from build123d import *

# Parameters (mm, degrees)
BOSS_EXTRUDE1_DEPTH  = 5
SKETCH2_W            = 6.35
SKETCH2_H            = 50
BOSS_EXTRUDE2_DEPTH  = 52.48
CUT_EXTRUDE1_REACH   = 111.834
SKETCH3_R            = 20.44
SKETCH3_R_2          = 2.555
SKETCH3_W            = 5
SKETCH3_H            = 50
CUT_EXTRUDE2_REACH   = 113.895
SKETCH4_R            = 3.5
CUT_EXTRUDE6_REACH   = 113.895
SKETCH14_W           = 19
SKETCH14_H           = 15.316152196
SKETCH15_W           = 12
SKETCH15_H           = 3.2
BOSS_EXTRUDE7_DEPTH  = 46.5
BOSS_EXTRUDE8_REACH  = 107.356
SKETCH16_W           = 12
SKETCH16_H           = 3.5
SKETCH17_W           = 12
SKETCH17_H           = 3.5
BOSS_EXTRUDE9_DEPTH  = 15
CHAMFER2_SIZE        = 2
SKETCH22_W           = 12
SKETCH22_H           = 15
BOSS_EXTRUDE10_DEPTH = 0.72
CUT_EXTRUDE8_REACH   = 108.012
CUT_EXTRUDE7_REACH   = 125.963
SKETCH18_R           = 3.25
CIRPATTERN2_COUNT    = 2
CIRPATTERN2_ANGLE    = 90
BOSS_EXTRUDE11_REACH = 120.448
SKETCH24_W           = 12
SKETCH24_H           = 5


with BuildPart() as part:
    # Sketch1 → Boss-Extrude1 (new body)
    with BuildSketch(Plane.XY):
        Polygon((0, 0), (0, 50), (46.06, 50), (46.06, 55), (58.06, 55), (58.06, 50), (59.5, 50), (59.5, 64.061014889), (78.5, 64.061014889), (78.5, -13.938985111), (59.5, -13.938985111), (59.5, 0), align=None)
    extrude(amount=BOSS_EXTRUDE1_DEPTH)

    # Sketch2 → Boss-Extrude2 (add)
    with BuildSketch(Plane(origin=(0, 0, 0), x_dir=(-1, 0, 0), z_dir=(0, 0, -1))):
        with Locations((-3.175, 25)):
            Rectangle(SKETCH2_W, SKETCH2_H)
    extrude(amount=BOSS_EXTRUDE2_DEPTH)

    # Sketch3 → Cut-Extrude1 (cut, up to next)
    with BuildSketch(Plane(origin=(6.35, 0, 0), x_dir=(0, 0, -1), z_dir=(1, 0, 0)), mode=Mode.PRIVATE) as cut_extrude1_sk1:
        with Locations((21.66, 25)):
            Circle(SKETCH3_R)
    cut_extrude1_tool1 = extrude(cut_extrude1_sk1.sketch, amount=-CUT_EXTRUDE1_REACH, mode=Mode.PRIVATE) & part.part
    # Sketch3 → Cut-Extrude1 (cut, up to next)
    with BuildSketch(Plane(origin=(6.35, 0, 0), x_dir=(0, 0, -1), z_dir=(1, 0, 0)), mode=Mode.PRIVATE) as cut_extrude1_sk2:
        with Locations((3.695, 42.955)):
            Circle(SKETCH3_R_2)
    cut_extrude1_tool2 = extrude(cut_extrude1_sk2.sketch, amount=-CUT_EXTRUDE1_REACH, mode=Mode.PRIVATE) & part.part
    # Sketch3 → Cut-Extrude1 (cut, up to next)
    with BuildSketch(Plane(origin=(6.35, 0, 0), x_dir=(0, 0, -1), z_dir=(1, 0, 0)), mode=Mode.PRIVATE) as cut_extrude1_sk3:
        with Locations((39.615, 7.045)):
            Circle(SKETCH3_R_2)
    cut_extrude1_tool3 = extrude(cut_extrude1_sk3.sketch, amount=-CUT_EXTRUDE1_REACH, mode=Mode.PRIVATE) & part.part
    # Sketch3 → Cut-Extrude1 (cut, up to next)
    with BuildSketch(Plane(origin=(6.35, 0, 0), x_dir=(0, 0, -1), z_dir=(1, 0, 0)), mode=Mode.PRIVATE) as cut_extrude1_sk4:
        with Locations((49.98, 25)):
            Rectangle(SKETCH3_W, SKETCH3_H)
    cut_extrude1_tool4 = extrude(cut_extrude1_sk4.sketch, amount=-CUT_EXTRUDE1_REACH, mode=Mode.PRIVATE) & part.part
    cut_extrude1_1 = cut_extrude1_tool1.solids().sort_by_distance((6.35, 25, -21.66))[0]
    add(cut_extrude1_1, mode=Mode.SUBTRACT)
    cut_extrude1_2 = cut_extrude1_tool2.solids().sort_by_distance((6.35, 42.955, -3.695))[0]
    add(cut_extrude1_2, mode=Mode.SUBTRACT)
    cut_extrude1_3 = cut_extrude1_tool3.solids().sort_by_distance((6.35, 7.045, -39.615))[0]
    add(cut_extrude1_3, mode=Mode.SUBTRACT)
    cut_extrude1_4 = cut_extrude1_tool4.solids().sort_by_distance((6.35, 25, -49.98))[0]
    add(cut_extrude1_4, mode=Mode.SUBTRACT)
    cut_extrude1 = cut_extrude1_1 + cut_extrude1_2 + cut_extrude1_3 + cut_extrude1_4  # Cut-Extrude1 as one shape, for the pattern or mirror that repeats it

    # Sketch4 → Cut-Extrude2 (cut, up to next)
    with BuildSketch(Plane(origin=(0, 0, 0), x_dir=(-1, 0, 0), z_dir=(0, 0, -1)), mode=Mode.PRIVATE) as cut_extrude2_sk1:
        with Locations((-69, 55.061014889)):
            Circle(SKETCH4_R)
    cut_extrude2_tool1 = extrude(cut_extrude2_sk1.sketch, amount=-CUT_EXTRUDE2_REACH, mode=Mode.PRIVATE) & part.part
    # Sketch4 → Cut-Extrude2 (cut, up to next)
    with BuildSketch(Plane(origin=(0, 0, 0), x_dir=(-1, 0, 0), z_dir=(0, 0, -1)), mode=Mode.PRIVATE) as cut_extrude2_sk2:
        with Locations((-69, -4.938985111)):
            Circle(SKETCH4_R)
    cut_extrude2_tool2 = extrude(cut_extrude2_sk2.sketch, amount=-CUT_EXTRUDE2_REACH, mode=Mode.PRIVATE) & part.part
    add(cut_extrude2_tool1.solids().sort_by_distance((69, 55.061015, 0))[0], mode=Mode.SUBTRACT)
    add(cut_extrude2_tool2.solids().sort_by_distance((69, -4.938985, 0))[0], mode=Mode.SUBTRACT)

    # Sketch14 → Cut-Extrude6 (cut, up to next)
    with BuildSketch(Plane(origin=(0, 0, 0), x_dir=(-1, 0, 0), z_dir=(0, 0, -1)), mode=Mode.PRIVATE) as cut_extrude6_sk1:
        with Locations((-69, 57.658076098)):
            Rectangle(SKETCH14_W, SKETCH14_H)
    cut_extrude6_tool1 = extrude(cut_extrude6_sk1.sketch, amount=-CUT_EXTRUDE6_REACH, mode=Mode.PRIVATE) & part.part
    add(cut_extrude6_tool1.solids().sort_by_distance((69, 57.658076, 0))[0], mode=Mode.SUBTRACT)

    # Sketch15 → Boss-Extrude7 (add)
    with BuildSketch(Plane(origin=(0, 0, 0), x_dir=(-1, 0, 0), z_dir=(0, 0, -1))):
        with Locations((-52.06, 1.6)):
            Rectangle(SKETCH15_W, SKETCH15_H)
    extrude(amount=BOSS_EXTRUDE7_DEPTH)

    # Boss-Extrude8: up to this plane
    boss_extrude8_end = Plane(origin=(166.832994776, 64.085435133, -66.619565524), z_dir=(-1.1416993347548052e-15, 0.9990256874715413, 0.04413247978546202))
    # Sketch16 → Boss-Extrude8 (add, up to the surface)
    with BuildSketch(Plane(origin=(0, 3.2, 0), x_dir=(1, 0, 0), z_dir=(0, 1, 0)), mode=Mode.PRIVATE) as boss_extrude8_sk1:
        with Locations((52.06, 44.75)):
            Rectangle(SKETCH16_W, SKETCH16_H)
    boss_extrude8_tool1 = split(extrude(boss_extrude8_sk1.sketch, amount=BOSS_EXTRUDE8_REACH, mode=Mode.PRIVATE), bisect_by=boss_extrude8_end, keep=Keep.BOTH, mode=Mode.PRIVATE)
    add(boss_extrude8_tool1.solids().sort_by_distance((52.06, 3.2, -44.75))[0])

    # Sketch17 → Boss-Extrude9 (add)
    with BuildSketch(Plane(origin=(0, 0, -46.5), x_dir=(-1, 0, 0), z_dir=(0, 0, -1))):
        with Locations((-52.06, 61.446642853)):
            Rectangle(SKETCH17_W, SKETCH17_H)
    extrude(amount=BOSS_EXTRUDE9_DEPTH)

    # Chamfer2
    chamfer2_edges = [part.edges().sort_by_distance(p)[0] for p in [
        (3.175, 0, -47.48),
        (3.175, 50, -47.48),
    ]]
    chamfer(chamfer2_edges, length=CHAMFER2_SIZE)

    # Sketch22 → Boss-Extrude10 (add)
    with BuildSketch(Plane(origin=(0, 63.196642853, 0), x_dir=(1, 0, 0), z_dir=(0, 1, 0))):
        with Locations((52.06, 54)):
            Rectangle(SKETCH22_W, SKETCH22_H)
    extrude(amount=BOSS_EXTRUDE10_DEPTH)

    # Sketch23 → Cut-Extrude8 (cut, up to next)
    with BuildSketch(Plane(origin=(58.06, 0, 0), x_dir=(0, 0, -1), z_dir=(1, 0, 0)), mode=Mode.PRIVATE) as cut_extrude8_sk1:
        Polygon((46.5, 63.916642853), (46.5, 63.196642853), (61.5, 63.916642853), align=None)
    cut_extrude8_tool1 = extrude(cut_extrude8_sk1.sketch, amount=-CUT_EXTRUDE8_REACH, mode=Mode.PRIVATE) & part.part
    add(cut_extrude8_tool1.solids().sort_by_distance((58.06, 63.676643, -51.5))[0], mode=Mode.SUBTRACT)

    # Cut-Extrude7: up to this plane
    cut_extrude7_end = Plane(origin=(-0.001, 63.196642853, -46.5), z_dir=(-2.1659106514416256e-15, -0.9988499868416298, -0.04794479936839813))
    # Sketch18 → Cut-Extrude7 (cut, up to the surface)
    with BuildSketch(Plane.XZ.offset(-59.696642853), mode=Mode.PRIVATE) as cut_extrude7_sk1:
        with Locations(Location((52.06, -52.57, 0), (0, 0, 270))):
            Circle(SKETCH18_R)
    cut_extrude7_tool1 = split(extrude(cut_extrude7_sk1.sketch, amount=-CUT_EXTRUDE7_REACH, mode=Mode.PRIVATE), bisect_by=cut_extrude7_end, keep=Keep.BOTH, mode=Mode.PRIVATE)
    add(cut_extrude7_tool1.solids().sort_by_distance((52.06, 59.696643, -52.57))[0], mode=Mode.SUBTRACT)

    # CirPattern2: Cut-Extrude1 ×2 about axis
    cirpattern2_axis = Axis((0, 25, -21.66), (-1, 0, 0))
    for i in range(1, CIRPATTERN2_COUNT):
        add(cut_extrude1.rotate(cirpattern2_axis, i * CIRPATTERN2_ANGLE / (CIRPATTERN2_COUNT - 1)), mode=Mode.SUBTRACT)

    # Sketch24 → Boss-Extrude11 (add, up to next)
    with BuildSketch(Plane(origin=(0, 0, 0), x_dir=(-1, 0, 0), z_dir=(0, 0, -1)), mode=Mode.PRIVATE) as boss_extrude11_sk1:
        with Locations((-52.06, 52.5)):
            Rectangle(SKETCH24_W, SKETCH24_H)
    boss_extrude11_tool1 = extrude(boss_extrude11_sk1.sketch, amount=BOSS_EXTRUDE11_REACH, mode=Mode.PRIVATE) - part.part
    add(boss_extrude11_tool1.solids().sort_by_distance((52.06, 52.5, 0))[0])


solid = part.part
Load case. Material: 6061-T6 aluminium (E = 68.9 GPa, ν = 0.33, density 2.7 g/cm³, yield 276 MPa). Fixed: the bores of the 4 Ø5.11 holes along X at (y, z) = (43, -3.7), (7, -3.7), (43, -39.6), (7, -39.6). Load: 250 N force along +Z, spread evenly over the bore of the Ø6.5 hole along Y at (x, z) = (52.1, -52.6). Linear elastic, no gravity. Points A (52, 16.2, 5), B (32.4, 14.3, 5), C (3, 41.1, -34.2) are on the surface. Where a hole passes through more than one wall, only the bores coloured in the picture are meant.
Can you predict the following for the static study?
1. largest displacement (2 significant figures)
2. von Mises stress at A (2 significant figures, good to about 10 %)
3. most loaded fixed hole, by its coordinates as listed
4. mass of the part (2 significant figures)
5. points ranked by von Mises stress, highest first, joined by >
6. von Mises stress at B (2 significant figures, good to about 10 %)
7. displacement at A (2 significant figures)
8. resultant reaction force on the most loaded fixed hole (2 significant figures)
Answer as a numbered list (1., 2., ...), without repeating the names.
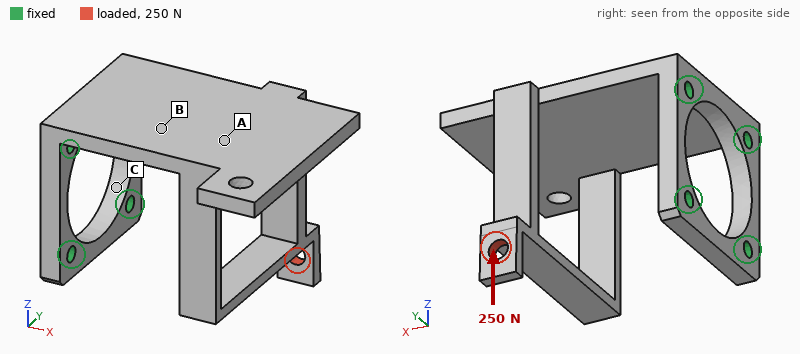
1. 1.1 mm
2. 16 MPa
3. (43, -3.7)
4. 94 g
5. B > A > C
6. 36 MPa
7. 0.27 mm
8. 370 N
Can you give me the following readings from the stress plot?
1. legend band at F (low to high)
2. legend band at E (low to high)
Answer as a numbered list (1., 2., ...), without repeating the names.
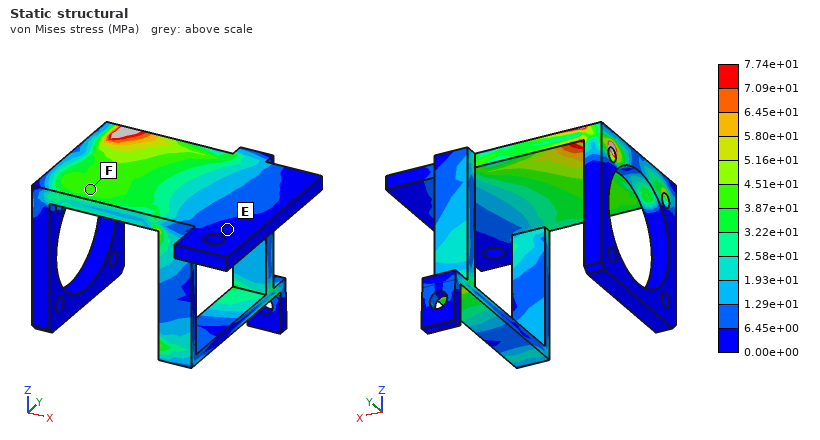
1. 3.87e+01 to 4.51e+01 MPa
2. 0.00e+00 to 6.45e+00 MPa
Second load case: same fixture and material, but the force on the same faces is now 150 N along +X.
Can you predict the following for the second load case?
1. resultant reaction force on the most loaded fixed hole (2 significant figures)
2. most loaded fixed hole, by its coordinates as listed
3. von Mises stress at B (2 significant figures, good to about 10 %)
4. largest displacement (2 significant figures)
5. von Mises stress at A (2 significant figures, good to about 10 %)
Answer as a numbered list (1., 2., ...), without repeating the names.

1. 230 N
2. (43, -3.7)
3. 36 MPa
4. 1.3 mm
5. 19 MPa
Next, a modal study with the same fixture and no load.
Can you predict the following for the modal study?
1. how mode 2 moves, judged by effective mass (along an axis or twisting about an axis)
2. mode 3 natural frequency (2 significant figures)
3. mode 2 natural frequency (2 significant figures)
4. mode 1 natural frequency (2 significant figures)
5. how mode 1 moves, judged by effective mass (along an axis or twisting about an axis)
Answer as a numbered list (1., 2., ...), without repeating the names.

1. along Y
2. 1300 Hz
3. 710 Hz
4. 440 Hz
5. along Z
